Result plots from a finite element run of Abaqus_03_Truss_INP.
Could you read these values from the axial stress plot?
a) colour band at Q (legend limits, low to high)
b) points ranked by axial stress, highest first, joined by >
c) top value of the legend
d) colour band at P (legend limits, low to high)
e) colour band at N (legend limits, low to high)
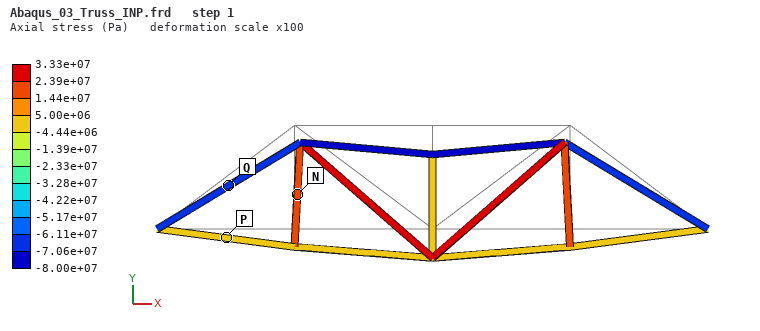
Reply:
-7.06e+07 to -6.11e+07 Pa
N > P > Q
3.33e+07 Pa
-4.44e+06 to 5.00e+06 Pa
1.44e+07 to 2.39e+07 Pa
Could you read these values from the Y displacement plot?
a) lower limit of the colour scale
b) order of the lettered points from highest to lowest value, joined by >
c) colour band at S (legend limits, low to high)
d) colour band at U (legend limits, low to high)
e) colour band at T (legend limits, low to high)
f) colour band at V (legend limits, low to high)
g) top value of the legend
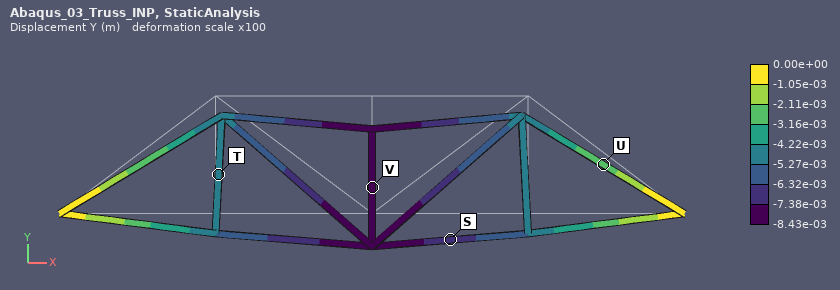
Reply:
-8.43e-03 m
U > T > S > V
-7.38e-03 to -6.32e-03 m
-3.16e-03 to -2.11e-03 m
-5.27e-03 to -4.22e-03 m
-8.43e-03 to -7.38e-03 m
0.00e+00 m
